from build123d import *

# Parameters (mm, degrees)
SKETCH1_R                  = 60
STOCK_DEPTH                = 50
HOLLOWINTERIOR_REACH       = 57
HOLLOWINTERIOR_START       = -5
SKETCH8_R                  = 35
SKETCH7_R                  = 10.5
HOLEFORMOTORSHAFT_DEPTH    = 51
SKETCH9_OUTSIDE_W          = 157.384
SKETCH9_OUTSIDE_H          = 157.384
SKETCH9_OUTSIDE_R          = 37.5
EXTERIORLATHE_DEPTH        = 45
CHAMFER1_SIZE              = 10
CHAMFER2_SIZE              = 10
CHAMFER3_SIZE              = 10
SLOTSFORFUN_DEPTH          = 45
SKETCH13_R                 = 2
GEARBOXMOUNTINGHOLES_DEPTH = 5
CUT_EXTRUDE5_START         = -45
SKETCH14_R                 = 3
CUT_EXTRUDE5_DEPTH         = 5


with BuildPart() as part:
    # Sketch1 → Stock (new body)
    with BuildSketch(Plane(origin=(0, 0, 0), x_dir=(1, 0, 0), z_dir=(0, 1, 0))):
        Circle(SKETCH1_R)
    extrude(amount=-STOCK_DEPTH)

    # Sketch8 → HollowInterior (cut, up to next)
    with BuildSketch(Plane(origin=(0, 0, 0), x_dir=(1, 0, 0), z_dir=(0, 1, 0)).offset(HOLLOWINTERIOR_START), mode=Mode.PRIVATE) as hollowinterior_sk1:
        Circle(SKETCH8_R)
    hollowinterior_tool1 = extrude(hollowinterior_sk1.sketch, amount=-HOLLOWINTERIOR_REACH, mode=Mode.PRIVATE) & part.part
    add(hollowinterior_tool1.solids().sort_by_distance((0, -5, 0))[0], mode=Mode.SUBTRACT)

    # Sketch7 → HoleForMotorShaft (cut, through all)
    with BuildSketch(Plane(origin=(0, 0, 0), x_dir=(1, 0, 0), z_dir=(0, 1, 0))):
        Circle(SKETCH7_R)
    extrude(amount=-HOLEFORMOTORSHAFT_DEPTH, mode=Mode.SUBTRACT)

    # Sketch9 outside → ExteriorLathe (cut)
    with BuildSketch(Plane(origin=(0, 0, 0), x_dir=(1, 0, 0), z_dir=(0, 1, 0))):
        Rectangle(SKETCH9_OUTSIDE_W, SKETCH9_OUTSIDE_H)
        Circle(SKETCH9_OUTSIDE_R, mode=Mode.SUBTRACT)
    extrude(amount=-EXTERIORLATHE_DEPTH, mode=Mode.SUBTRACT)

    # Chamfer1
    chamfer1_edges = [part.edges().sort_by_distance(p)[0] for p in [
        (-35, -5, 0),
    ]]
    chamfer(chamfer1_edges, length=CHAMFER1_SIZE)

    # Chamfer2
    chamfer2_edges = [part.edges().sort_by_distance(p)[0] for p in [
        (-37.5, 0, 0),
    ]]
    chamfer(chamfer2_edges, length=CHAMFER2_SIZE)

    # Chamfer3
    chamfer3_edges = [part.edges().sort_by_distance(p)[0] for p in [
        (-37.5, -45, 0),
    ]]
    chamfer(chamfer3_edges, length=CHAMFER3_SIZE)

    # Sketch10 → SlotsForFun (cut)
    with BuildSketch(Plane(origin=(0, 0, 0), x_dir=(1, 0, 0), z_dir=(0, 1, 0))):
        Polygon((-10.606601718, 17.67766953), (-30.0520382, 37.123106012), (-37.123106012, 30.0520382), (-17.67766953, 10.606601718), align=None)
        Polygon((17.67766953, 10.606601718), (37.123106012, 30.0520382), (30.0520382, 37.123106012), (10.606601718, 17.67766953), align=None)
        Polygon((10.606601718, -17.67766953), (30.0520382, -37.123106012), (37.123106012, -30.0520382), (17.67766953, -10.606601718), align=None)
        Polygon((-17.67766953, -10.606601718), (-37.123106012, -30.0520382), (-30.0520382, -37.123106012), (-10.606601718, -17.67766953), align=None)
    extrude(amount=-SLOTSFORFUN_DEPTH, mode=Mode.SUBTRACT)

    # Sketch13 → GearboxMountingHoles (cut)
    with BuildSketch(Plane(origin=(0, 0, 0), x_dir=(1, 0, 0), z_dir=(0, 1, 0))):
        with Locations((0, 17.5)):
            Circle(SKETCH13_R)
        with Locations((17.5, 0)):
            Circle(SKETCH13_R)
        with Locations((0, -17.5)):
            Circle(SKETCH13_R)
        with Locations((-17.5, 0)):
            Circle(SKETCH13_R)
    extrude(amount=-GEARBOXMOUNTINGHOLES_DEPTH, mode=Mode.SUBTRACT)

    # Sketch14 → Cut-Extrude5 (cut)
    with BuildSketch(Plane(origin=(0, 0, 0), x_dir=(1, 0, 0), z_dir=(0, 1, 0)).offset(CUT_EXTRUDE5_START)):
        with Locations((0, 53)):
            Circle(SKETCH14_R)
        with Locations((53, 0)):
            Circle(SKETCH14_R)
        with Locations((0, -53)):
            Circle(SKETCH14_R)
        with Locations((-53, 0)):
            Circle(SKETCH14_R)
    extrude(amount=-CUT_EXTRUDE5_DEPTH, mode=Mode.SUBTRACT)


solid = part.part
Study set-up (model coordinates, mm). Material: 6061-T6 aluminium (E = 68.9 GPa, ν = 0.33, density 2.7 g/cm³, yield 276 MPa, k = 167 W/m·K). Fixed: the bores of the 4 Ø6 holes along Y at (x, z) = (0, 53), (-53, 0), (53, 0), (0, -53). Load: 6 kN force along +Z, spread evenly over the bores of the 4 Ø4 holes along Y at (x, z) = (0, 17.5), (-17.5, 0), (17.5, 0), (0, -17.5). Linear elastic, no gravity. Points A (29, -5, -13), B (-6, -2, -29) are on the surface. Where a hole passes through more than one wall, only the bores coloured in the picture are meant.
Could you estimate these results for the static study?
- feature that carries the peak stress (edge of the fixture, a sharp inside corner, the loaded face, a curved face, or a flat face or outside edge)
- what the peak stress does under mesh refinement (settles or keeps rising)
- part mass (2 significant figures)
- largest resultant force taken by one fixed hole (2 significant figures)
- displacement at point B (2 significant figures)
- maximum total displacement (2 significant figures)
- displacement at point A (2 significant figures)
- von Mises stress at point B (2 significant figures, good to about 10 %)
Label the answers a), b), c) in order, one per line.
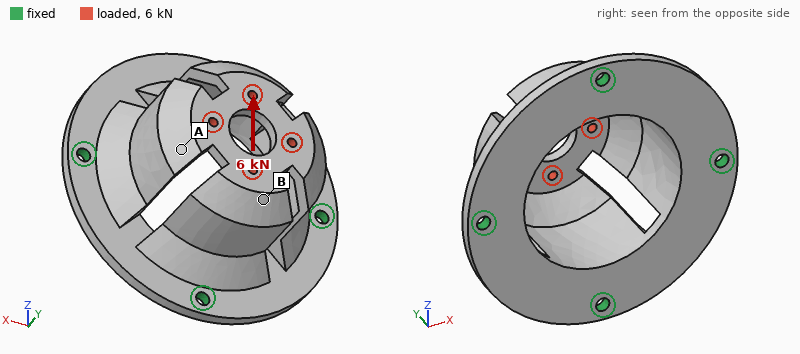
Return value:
a) edge of the fixture
b) keeps rising
c) 220 g
d) 3.1 kN
e) 0.21 mm
f) 0.21 mm
g) 0.18 mm
h) 35 MPa
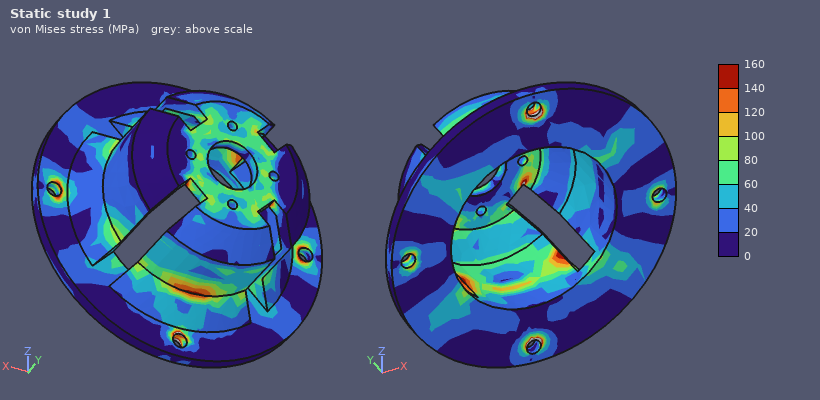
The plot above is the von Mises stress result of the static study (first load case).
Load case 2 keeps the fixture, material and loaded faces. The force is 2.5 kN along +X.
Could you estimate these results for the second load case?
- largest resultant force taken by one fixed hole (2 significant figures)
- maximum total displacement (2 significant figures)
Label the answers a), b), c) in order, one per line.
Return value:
a) 1.3 kN
b) 89 µm
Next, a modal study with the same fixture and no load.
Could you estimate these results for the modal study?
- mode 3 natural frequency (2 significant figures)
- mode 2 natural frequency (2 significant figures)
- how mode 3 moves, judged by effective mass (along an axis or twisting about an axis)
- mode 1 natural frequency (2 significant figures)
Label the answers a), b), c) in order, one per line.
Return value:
a) 4600 Hz
b) 3600 Hz
c) along Y
d) 3500 Hz
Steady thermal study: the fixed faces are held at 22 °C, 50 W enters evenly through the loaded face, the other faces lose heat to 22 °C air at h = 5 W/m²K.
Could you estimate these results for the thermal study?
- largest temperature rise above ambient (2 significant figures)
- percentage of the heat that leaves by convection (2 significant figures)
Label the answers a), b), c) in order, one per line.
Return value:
a) 35 K
b) 4.8 %
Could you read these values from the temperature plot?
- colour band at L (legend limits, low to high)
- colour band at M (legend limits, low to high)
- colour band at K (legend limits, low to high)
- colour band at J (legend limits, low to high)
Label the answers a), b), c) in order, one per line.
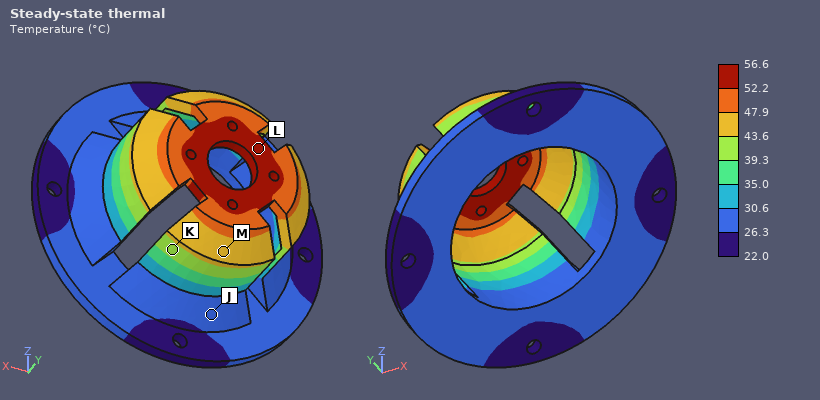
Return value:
a) 52.2 to 56.6 °C
b) 43.6 to 47.9 °C
c) 39.3 to 43.6 °C
d) 26.3 to 30.6 °C
